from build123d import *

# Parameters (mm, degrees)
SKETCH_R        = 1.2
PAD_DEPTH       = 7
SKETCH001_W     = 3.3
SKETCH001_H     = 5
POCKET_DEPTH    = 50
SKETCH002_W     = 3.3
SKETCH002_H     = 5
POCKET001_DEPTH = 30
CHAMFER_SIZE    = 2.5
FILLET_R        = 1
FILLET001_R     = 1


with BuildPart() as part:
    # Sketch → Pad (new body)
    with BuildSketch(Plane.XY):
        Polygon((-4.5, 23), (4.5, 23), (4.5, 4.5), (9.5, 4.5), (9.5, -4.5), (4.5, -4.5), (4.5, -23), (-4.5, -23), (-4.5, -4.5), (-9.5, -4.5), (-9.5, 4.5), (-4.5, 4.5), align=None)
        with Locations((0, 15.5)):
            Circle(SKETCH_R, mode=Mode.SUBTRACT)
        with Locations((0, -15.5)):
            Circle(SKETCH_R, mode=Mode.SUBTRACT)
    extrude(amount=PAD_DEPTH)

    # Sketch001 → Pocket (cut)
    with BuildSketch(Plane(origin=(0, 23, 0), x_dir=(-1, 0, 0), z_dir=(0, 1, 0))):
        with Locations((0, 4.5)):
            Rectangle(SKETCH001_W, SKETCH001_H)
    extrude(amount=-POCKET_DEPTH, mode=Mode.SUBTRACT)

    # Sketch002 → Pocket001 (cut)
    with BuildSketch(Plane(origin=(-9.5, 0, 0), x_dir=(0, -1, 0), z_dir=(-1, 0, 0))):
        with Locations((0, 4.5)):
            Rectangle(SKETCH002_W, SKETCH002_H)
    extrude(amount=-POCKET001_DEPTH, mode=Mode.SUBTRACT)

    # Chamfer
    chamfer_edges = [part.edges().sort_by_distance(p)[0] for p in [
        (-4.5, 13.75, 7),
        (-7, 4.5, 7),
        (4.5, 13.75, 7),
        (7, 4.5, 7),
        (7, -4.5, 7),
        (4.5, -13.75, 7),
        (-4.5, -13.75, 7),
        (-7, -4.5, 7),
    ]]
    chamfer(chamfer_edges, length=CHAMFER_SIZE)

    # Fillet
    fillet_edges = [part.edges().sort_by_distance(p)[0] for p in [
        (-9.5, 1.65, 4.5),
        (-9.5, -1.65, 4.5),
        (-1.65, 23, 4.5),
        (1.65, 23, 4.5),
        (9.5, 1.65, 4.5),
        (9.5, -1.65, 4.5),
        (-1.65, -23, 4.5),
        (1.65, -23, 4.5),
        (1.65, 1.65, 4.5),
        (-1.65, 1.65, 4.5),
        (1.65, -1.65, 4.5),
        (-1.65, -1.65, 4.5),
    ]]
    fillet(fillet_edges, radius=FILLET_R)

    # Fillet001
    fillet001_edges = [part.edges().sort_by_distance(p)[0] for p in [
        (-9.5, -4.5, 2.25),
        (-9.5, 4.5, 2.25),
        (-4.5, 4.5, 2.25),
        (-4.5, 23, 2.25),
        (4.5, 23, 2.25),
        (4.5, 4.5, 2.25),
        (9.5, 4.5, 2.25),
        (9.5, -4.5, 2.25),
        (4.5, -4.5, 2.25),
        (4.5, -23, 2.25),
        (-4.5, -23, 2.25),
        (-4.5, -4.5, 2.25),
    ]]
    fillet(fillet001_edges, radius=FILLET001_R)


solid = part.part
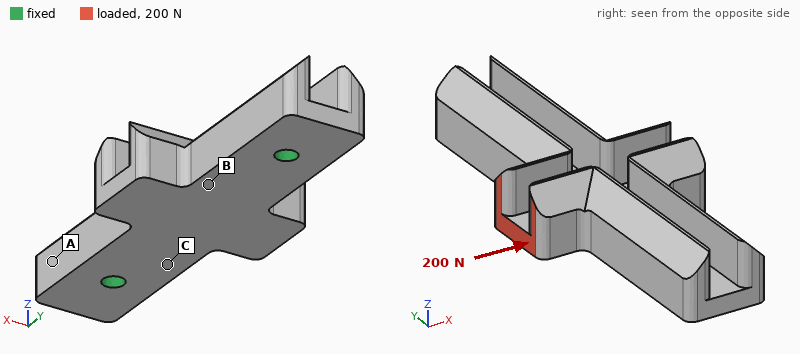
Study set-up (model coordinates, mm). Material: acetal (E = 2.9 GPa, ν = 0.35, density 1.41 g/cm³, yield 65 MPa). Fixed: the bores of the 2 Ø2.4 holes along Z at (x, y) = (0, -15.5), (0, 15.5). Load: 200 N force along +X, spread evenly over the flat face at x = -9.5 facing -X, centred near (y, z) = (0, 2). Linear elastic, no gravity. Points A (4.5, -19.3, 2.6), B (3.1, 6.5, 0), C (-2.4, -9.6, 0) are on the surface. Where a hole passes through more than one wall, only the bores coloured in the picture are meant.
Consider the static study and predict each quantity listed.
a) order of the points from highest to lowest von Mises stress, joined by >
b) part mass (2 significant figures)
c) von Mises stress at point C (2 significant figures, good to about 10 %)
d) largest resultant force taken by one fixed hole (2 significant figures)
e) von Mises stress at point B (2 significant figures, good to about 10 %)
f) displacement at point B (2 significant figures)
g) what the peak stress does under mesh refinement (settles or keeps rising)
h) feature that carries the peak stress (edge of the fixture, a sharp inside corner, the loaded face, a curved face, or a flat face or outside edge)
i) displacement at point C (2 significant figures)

B > C > A
3.0 g
6.7 MPa
100 N
11 MPa
0.099 mm
keeps rising
edge of the fixture
0.063 mm
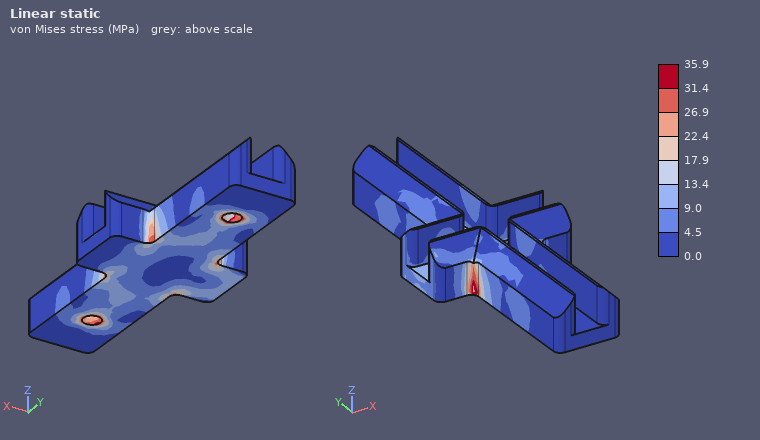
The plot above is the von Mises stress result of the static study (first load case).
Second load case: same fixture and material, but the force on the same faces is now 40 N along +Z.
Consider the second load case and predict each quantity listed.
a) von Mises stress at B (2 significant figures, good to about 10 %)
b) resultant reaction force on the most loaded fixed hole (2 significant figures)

5.4 MPa
20 N
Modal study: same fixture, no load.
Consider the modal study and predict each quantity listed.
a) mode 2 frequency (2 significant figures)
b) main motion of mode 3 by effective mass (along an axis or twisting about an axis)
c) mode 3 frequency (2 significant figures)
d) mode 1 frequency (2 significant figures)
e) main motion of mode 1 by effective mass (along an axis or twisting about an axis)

2800 Hz
along X
5200 Hz
2600 Hz
along Z
